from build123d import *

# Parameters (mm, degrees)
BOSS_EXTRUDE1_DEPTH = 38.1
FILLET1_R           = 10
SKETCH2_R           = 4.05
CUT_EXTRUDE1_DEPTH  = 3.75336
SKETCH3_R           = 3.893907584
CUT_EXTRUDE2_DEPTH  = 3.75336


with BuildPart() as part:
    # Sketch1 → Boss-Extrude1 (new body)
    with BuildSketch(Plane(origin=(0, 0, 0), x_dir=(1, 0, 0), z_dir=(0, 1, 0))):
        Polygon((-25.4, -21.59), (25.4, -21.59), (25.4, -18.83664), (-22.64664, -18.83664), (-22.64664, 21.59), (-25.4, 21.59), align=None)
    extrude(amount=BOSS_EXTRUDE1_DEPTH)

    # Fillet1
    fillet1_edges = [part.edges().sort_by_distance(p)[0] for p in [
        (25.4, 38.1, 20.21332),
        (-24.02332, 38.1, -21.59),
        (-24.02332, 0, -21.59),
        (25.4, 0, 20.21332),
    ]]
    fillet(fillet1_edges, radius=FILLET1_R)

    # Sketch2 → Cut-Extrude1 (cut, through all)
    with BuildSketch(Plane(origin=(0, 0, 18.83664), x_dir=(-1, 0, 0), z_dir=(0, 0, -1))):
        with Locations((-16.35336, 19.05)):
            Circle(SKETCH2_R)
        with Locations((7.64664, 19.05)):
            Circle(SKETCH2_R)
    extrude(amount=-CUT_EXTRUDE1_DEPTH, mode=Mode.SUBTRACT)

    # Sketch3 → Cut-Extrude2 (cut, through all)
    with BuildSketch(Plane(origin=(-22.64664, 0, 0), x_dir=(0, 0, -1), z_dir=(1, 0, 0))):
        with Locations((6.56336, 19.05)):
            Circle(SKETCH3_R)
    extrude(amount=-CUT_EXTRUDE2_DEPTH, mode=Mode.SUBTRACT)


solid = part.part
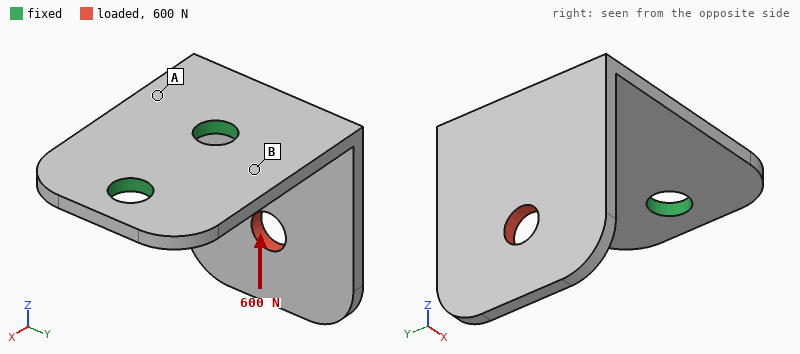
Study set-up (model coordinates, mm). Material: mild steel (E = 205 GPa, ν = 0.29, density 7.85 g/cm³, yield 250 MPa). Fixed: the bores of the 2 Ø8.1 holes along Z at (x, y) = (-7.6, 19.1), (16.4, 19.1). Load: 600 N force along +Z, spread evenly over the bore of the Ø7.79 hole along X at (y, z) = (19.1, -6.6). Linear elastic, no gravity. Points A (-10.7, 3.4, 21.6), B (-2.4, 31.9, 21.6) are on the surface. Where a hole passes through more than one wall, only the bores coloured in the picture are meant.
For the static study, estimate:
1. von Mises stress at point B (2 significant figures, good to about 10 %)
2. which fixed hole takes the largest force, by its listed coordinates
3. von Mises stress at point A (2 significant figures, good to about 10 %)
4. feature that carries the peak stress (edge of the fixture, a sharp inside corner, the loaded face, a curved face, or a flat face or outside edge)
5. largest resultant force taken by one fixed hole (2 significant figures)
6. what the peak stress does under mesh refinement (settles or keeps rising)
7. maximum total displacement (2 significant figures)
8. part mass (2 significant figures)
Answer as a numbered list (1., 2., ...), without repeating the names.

1. 28 MPa
2. (-7.6, 19.1)
3. 69 MPa
4. edge of the fixture
5. 660 N
6. keeps rising
7. 0.21 mm
8. 70 g
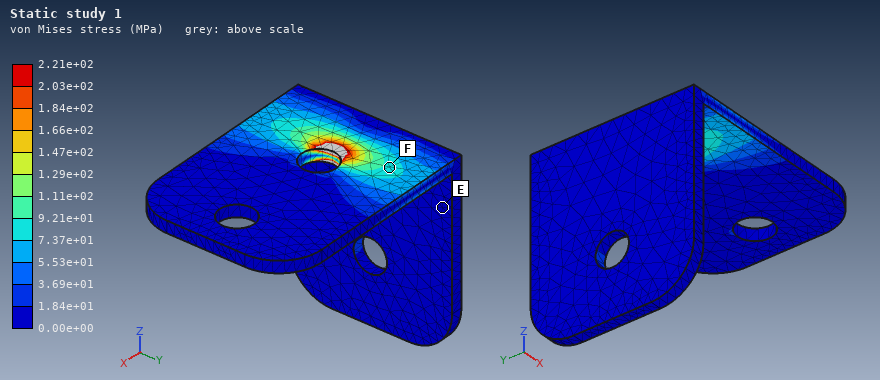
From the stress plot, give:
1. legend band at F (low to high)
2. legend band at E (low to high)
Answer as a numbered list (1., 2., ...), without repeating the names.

1. 7.37e+01 to 9.21e+01 MPa
2. 0.00e+00 to 1.84e+01 MPa
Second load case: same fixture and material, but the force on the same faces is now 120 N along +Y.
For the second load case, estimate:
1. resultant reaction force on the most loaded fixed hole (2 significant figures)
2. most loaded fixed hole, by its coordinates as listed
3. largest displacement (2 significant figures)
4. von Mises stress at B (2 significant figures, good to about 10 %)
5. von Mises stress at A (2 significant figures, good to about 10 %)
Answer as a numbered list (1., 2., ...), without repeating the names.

1. 170 N
2. (-7.6, 19.1)
3. 71 µm
4. 24 MPa
5. 27 MPa
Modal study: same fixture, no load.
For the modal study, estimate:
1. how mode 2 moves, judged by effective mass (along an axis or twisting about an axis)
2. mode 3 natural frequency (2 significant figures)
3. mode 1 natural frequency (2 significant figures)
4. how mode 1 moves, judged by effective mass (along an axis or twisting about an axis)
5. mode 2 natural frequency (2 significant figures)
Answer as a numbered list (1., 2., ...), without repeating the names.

1. along Y
2. 3400 Hz
3. 900 Hz
4. along X
5. 1500 Hz
